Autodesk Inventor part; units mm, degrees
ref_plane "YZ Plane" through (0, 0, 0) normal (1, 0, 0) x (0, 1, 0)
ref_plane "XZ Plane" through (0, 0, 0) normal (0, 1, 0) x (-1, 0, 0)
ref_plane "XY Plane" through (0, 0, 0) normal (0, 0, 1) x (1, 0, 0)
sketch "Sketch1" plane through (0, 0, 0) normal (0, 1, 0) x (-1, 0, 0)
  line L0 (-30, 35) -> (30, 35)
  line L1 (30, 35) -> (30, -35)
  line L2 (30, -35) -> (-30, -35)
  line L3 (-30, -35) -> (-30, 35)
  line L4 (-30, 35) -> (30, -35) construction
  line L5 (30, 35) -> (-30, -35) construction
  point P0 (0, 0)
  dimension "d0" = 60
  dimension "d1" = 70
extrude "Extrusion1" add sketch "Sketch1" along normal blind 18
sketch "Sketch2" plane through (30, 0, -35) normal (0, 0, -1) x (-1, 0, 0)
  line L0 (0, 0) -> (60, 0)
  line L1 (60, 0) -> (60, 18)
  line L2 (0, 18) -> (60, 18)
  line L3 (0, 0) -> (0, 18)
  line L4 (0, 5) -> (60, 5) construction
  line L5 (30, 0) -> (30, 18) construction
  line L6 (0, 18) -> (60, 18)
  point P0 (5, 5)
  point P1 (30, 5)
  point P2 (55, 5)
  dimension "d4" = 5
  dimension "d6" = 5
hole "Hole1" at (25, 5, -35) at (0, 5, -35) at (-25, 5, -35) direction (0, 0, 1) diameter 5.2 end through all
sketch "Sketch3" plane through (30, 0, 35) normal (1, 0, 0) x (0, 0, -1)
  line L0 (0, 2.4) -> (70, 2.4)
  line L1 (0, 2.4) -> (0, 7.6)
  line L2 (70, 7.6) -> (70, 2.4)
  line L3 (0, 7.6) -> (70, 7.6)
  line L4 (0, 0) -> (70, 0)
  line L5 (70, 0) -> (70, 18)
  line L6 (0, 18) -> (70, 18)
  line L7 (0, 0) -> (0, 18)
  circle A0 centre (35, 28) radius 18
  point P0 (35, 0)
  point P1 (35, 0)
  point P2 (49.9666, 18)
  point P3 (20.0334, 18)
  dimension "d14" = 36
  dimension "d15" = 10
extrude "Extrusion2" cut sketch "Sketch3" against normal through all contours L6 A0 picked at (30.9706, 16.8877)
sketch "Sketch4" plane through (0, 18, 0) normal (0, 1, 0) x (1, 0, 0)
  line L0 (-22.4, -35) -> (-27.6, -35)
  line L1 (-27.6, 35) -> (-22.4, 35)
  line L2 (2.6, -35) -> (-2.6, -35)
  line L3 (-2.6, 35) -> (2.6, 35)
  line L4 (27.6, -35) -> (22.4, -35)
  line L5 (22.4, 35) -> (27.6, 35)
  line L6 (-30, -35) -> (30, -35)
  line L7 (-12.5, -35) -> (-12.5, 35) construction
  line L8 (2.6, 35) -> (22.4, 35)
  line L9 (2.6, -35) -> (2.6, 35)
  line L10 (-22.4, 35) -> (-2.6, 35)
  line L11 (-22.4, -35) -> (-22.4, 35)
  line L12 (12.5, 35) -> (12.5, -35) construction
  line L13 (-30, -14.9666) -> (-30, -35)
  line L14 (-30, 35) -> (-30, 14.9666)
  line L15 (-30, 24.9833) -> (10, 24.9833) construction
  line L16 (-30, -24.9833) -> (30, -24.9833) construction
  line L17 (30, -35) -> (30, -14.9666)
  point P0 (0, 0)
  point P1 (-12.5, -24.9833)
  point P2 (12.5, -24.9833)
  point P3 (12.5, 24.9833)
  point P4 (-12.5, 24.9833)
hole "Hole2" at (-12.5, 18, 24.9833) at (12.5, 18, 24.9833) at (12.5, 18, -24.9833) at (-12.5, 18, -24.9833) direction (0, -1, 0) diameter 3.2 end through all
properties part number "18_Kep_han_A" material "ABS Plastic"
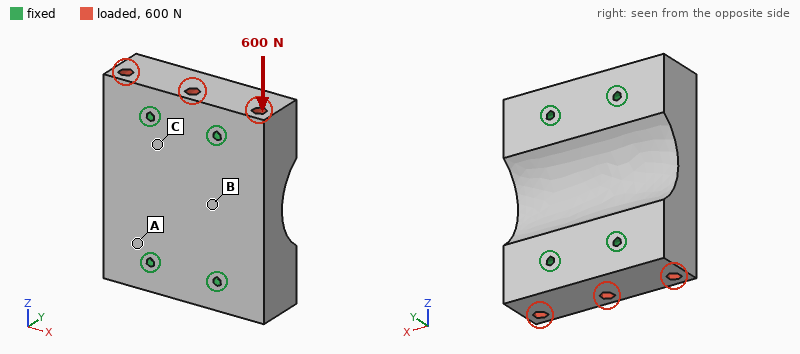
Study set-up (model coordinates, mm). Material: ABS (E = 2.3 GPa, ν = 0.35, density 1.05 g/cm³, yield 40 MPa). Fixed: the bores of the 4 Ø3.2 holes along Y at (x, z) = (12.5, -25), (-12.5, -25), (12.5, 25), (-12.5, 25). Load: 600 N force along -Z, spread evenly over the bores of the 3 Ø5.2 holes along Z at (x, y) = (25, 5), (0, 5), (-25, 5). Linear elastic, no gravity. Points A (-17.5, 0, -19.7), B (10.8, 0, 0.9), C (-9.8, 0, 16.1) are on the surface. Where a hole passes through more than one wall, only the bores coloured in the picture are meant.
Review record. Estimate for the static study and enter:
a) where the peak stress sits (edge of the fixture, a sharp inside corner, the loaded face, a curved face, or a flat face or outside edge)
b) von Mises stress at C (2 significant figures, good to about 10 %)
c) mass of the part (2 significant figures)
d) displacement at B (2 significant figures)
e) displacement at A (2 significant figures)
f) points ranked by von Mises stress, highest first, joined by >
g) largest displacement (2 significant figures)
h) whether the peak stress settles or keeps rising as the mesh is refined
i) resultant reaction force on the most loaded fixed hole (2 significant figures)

edge of the fixture
0.31 MPa
63 g
2.8 µm
3.0 µm
A > C > B
8.5 µm
keeps rising
150 N
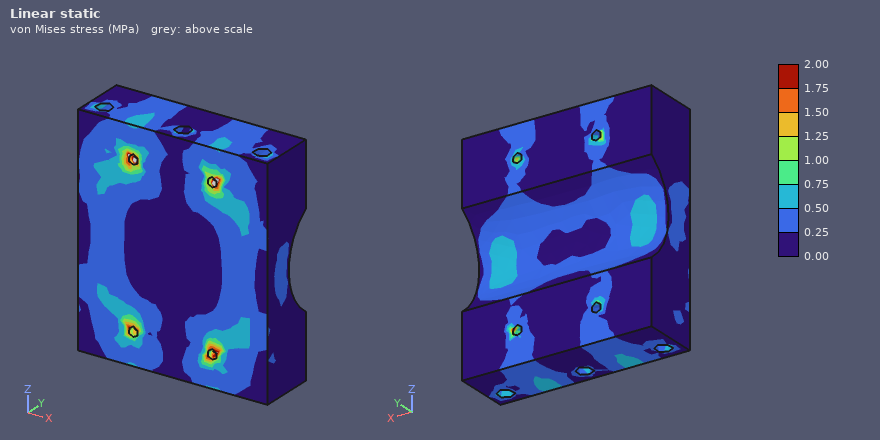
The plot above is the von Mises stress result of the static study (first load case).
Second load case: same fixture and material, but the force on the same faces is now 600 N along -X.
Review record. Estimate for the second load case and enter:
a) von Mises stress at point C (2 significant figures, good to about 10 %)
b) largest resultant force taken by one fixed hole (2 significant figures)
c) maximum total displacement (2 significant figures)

0.45 MPa
150 N
10 µm
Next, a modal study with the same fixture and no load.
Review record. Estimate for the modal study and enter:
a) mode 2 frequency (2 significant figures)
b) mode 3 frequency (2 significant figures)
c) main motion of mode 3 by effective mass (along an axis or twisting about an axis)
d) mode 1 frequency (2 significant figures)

5400 Hz
7500 Hz
along X
5400 Hz
